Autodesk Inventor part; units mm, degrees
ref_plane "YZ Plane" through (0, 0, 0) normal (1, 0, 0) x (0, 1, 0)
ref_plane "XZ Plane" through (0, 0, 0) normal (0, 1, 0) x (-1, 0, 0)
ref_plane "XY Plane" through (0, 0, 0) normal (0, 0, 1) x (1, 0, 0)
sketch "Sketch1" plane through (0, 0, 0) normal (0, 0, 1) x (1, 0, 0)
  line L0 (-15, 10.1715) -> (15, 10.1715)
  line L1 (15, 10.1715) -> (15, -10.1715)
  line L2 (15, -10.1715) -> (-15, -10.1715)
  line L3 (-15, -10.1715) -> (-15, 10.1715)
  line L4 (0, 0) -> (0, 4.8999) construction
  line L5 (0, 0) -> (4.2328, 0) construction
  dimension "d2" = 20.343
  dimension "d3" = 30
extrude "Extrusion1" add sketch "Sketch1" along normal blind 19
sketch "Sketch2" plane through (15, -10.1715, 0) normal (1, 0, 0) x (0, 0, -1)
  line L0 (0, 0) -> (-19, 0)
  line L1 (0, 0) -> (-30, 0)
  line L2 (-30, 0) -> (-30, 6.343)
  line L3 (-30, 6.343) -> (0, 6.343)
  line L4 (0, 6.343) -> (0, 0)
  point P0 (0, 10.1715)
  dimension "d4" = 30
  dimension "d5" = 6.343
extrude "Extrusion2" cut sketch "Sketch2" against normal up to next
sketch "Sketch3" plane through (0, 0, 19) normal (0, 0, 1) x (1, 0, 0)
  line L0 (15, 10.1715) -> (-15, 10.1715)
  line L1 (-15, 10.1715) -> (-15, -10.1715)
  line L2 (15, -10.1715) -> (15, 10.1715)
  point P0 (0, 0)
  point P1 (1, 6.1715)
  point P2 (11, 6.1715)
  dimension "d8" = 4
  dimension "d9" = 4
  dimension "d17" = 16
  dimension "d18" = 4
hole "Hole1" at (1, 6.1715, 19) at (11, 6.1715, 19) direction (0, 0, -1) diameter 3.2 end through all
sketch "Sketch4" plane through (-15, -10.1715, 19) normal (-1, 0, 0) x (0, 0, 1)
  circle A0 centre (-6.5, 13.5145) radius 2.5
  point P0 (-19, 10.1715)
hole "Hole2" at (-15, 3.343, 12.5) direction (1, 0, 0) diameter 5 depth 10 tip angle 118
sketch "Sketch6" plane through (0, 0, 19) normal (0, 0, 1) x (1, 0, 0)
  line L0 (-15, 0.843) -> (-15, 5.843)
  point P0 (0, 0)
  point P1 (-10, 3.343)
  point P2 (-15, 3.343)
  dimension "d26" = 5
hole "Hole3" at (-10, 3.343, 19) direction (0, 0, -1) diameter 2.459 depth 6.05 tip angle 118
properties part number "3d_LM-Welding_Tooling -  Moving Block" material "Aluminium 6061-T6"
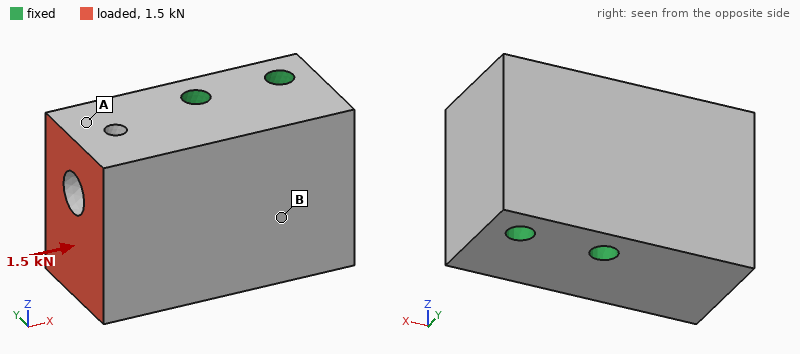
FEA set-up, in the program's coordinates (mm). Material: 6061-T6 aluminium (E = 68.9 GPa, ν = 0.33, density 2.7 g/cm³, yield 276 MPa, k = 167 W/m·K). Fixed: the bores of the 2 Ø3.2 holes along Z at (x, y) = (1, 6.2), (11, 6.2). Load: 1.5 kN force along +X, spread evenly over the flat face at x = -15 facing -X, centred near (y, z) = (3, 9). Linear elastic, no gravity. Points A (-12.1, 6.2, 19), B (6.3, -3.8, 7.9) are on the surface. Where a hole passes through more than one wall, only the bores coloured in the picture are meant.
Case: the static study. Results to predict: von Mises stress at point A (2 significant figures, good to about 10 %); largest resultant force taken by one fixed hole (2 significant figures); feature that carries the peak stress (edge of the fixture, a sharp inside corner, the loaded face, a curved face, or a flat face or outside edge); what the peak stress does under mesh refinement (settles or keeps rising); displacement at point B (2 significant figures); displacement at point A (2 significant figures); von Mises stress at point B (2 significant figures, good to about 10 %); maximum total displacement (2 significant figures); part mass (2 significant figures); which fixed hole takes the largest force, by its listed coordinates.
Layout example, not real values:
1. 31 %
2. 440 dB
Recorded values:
1. 7.7 MPa
2. 1.2 kN
3. edge of the fixture
4. keeps rising
5. 0.75 µm
6. 1.8 µm
7. 2.8 MPa
8. 3.1 µm
9. 20 g
10. (1, 6.2)
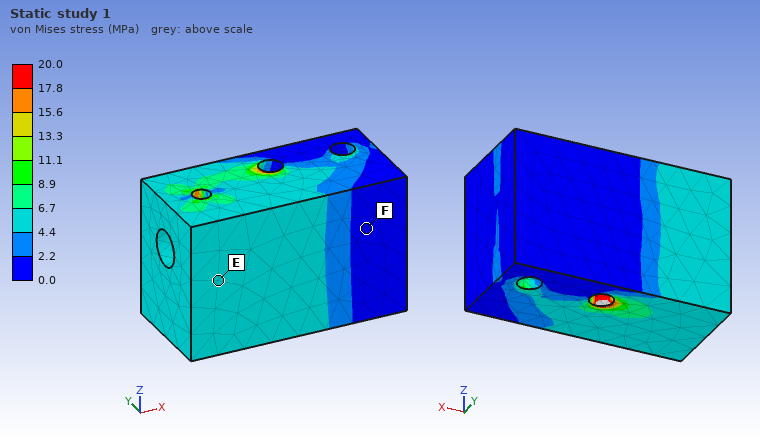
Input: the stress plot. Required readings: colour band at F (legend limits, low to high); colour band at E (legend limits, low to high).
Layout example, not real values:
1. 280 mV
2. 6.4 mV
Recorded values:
1. 0.0 to 2.2 MPa
2. 4.4 to 6.7 MPa
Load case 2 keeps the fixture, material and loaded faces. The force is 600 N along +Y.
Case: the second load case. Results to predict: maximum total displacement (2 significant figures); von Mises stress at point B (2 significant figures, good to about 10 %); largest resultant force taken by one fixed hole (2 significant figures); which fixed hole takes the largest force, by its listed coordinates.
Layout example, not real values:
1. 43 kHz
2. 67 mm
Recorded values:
1. 8.6 µm
2. 5.6 MPa
3. 1.2 kN
4. (1, 6.2)
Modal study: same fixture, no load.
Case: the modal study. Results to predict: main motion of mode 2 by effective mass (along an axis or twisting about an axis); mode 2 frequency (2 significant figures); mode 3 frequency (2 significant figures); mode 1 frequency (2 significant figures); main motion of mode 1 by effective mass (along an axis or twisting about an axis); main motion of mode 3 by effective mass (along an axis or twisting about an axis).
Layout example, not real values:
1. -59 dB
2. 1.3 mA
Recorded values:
1. along Z
2. 32 kHz
3. 41 kHz
4. 23 kHz
5. along Y
6. twisting about X
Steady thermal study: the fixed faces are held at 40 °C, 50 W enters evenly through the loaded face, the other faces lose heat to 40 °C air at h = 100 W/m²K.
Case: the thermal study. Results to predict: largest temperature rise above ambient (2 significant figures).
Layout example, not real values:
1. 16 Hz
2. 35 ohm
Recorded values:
1. 20 K
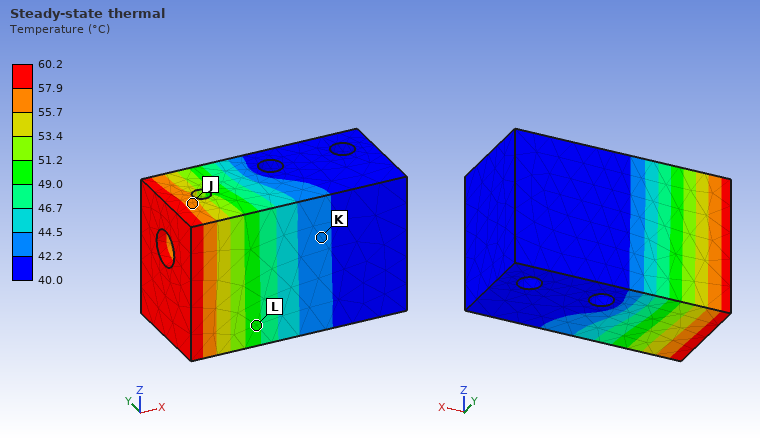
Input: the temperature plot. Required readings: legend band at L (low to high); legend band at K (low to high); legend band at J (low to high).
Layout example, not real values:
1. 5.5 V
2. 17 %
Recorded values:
1. 49.0 to 51.2 °C
2. 42.2 to 44.5 °C
3. 55.7 to 57.9 °C
